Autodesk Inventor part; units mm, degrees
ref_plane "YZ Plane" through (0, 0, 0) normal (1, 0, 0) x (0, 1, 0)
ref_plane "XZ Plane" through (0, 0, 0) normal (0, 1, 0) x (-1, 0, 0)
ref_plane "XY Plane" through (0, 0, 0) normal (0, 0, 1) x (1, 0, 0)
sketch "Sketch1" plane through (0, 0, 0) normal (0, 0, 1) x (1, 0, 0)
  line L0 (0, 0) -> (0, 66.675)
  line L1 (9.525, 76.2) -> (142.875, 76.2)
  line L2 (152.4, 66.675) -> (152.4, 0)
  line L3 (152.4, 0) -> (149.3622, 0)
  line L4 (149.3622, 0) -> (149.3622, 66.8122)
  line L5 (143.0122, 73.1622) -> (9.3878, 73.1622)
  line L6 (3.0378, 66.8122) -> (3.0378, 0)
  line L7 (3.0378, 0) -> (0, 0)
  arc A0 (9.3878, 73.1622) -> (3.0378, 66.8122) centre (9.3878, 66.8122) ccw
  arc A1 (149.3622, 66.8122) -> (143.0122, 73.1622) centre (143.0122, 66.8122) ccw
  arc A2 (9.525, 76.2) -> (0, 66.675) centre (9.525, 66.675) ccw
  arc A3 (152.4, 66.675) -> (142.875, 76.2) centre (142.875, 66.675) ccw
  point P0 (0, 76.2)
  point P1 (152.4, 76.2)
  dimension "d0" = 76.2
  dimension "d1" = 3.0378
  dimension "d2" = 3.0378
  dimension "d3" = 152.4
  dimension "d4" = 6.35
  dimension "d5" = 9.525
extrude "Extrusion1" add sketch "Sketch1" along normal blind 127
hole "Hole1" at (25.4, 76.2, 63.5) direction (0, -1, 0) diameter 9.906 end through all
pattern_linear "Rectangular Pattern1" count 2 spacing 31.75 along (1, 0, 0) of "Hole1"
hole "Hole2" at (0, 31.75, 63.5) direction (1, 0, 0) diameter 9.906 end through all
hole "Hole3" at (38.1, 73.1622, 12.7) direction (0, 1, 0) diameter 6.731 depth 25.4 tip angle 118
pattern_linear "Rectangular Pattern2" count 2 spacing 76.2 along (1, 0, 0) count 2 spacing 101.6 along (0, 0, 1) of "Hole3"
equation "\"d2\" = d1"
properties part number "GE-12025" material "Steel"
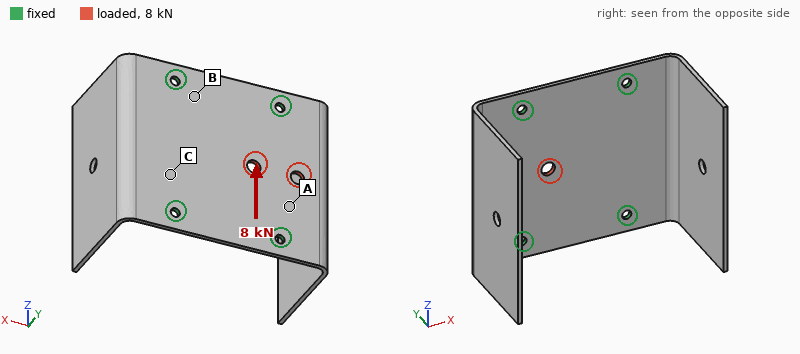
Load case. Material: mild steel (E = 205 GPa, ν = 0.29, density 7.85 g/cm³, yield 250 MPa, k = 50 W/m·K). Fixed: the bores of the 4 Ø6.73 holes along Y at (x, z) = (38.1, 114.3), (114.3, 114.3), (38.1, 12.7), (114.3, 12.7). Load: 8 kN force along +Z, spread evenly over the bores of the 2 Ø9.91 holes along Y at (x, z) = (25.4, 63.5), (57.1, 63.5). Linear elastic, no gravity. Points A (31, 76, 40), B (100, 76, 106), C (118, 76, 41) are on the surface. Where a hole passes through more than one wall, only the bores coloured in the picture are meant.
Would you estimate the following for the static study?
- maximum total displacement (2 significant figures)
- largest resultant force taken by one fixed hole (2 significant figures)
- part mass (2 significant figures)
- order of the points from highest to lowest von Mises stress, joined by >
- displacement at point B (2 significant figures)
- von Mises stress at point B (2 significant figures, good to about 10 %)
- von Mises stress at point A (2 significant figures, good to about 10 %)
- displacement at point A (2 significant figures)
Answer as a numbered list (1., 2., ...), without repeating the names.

1. 8.5 µm
2. 3.2 kN
3. 870 g
4. A > B > C
5. 1.4 µm
6. 13 MPa
7. 27 MPa
8. 4.9 µm
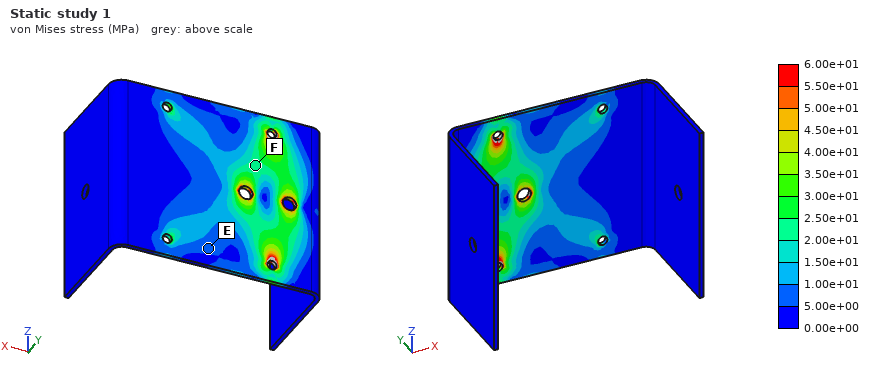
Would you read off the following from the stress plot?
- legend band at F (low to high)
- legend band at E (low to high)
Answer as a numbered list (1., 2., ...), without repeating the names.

1. 2.00e+01 to 2.50e+01 MPa
2. 5.00e+00 to 1.00e+01 MPa
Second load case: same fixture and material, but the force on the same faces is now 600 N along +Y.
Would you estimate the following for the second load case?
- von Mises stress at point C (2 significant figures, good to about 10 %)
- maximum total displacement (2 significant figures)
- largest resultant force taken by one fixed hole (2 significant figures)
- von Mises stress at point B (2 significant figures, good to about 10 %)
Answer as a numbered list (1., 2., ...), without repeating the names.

1. 8.2 MPa
2. 81 µm
3. 270 N
4. 11 MPa
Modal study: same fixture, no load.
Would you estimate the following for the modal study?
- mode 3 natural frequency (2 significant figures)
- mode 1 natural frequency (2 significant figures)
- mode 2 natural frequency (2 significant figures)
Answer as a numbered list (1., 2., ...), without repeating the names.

1. 520 Hz
2. 250 Hz
3. 250 Hz
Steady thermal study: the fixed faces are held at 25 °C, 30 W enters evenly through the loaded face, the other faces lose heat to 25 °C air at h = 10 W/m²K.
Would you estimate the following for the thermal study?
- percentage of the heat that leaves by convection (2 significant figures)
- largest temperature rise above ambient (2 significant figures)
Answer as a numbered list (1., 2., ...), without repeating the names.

1. 34 %
2. 63 K
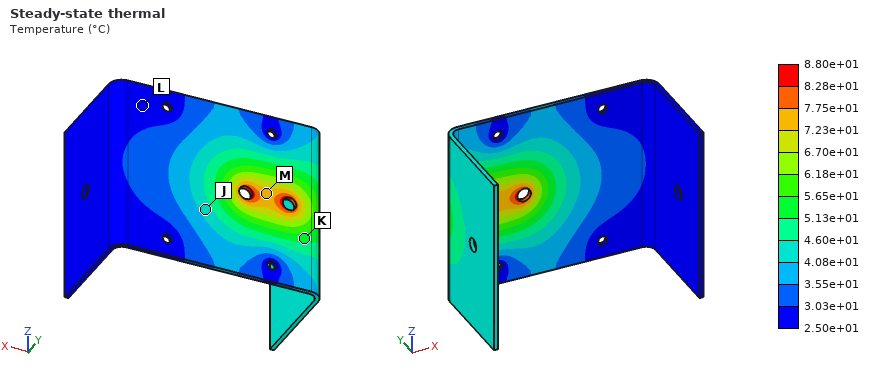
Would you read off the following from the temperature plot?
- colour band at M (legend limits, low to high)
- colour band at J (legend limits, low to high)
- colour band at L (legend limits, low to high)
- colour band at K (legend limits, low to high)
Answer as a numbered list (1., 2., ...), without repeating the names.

1. 7.23e+01 to 7.75e+01 °C
2. 4.08e+01 to 4.60e+01 °C
3. 2.50e+01 to 3.03e+01 °C
4. 5.13e+01 to 5.65e+01 °C
